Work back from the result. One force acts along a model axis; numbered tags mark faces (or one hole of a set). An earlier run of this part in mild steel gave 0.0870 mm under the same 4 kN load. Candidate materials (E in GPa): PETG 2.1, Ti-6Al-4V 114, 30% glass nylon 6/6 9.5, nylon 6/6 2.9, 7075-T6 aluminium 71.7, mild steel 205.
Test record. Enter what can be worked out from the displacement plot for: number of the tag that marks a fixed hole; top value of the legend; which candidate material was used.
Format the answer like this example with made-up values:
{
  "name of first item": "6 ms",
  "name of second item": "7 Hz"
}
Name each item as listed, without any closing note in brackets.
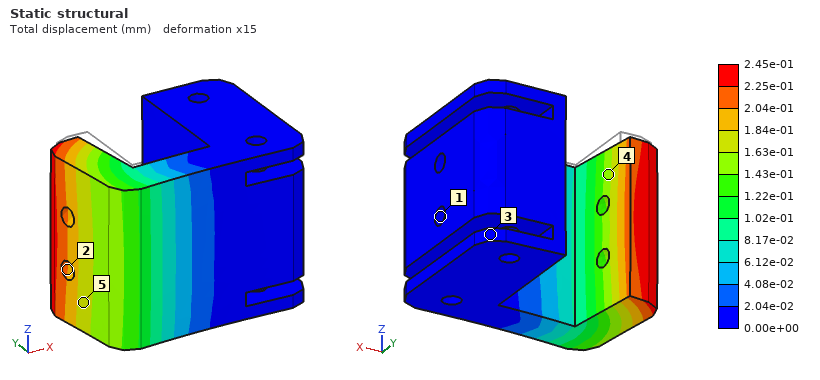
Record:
{
  "number of the tag that marks a fixed hole": "1",
  "top value of the legend": "2.45e-01 mm",
  "which candidate material was used": "7075-T6 aluminium"
}
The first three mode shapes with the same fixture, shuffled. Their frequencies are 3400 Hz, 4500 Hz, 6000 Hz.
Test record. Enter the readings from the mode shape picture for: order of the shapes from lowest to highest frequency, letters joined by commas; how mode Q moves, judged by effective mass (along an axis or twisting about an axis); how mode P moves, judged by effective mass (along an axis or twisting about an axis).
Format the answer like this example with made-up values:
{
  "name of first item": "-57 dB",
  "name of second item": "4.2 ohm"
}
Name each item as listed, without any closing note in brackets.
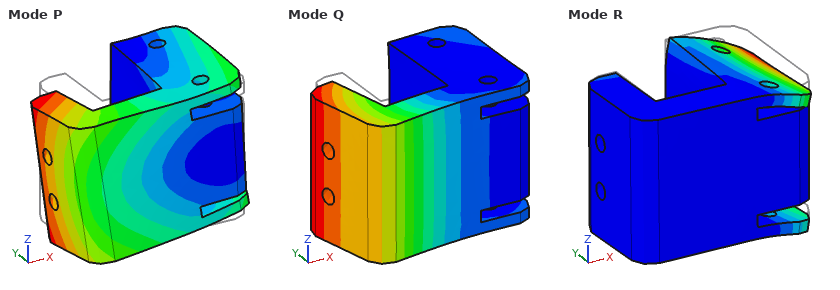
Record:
{
  "order of the shapes from lowest to highest frequency, letters joined by commas": "Q, P, R",
  "how mode Q moves, judged by effective mass": "along Y",
  "how mode P moves, judged by effective mass": "along Z"
}
